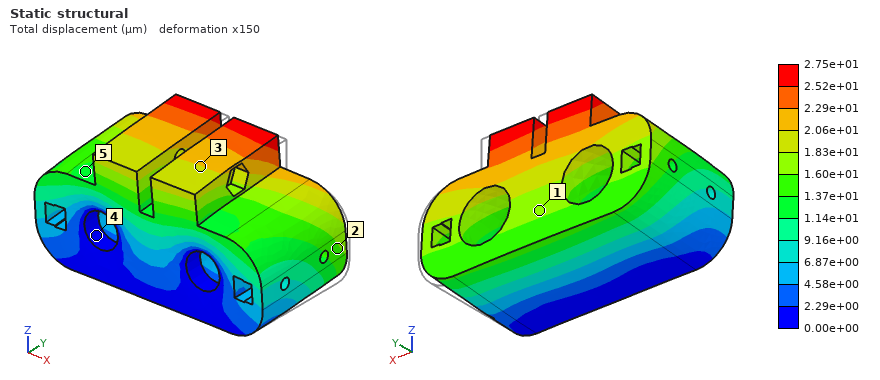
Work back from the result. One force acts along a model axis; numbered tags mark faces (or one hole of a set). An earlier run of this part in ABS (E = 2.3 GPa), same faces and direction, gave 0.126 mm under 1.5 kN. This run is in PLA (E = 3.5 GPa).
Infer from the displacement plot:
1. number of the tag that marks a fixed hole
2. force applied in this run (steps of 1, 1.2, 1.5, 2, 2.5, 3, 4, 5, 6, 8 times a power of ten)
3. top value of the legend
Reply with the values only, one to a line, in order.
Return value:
4
500 N
2.75e+01 µm
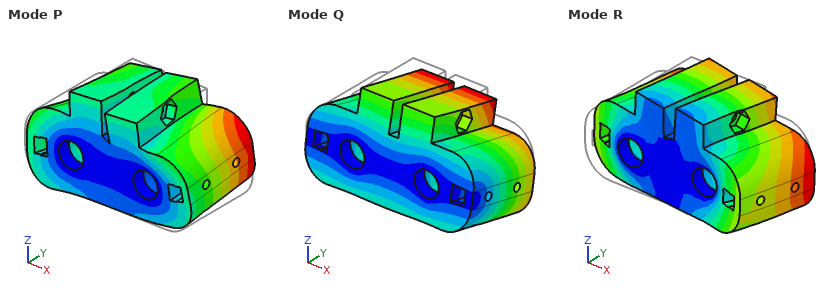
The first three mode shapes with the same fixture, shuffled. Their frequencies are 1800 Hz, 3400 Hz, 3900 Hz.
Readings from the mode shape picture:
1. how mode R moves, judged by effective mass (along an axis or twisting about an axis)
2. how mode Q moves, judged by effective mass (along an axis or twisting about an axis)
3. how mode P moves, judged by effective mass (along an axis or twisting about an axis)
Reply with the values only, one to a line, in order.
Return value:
along X
along Z
twisting about Y
